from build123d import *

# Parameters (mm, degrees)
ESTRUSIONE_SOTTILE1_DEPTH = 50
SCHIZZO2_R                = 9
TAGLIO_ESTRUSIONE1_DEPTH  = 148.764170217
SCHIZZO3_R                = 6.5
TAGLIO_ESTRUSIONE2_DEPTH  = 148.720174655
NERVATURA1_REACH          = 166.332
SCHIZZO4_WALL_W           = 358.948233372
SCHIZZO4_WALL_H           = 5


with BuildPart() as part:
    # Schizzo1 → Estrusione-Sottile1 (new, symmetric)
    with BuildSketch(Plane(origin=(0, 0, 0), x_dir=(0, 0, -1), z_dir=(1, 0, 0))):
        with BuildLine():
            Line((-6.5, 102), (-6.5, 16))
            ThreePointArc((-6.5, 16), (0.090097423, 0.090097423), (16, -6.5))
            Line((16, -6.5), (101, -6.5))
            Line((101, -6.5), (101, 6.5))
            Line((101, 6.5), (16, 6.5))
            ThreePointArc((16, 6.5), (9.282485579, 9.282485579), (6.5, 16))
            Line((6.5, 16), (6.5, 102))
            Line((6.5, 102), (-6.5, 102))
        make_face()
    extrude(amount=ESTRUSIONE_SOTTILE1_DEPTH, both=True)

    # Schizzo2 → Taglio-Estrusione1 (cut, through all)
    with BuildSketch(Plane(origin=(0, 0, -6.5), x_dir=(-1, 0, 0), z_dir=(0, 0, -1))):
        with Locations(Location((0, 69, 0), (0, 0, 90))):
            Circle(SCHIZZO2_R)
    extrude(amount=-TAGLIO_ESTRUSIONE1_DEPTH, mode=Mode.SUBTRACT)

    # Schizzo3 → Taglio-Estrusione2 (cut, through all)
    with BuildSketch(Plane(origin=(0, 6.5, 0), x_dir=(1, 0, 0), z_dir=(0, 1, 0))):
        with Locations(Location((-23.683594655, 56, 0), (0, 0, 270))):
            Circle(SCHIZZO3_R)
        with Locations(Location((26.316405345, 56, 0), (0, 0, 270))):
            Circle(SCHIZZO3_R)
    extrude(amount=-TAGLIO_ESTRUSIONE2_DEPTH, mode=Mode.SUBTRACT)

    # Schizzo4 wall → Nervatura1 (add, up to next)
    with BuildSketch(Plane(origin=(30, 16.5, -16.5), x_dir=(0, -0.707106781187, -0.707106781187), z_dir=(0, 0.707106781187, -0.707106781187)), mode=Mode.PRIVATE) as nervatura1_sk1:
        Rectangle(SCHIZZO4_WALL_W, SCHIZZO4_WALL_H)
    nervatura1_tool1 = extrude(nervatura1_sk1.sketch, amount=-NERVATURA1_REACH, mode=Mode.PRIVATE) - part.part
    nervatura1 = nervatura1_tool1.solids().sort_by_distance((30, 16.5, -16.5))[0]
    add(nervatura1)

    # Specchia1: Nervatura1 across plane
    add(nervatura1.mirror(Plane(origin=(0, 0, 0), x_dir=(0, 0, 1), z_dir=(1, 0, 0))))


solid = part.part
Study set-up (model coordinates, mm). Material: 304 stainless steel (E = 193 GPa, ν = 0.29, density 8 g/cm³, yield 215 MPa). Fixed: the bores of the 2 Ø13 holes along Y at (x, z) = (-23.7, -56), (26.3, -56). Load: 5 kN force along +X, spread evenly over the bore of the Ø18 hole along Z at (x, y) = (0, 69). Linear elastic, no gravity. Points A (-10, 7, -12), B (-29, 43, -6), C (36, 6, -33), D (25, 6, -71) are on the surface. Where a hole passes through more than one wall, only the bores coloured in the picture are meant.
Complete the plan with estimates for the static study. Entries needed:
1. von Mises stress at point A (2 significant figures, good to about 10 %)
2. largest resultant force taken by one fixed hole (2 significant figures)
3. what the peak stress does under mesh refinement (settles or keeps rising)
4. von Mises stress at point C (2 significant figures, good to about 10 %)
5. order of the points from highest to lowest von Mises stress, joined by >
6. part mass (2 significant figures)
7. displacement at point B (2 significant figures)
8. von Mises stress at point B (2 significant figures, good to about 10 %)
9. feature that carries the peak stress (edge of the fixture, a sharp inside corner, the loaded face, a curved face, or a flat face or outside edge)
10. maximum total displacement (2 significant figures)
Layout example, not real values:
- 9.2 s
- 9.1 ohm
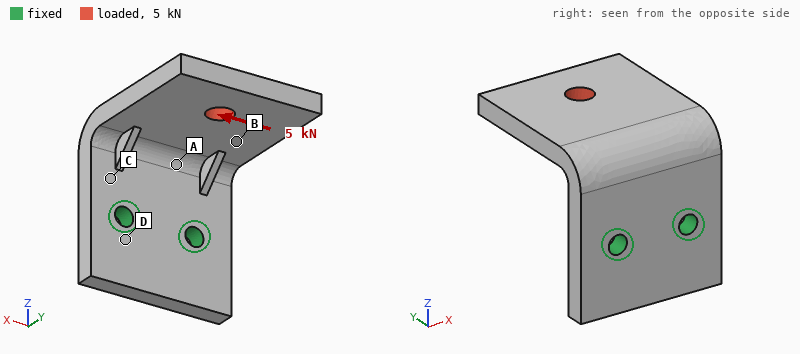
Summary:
- 77 MPa
- 7.4 kN
- keeps rising
- 54 MPa
- A > C > B > D
- 2.0 kg
- 0.093 mm
- 24 MPa
- edge of the fixture
- 0.20 mm
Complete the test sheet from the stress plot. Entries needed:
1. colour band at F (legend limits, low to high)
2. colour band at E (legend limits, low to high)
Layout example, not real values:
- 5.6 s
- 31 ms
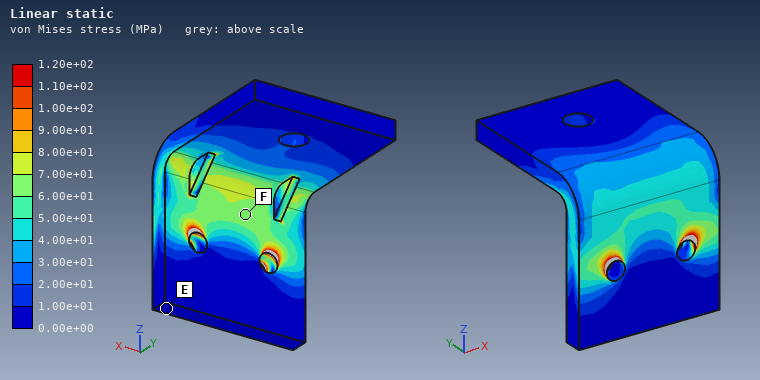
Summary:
- 6.00e+01 to 7.00e+01 MPa
- 0.00e+00 to 1.00e+01 MPa
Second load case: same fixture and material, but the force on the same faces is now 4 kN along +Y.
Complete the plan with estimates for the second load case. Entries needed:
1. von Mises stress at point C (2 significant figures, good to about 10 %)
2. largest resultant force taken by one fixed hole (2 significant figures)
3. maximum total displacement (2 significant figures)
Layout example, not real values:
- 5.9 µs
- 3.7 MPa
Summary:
- 45 MPa
- 2.1 kN
- 0.18 mm
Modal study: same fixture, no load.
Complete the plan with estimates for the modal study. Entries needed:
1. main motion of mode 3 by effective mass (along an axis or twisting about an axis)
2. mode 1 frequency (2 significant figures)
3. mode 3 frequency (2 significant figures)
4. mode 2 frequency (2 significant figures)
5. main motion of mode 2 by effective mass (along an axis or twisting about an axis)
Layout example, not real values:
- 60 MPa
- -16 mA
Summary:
- along Y
- 590 Hz
- 2000 Hz
- 1000 Hz
- along X
